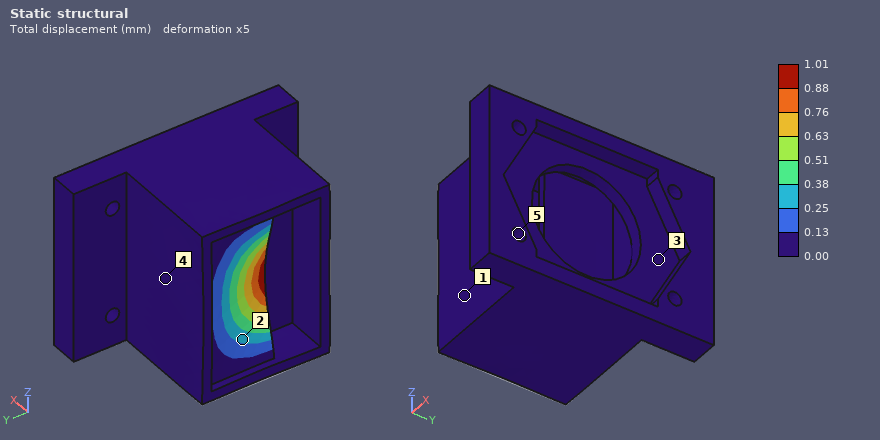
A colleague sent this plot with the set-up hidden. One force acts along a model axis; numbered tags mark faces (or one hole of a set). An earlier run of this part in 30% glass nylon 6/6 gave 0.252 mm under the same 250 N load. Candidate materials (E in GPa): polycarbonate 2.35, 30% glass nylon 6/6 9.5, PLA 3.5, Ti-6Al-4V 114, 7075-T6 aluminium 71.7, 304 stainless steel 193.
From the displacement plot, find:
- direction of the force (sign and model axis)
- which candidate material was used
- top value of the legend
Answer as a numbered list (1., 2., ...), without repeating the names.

1. +X
2. polycarbonate
3. 1.01 mm
